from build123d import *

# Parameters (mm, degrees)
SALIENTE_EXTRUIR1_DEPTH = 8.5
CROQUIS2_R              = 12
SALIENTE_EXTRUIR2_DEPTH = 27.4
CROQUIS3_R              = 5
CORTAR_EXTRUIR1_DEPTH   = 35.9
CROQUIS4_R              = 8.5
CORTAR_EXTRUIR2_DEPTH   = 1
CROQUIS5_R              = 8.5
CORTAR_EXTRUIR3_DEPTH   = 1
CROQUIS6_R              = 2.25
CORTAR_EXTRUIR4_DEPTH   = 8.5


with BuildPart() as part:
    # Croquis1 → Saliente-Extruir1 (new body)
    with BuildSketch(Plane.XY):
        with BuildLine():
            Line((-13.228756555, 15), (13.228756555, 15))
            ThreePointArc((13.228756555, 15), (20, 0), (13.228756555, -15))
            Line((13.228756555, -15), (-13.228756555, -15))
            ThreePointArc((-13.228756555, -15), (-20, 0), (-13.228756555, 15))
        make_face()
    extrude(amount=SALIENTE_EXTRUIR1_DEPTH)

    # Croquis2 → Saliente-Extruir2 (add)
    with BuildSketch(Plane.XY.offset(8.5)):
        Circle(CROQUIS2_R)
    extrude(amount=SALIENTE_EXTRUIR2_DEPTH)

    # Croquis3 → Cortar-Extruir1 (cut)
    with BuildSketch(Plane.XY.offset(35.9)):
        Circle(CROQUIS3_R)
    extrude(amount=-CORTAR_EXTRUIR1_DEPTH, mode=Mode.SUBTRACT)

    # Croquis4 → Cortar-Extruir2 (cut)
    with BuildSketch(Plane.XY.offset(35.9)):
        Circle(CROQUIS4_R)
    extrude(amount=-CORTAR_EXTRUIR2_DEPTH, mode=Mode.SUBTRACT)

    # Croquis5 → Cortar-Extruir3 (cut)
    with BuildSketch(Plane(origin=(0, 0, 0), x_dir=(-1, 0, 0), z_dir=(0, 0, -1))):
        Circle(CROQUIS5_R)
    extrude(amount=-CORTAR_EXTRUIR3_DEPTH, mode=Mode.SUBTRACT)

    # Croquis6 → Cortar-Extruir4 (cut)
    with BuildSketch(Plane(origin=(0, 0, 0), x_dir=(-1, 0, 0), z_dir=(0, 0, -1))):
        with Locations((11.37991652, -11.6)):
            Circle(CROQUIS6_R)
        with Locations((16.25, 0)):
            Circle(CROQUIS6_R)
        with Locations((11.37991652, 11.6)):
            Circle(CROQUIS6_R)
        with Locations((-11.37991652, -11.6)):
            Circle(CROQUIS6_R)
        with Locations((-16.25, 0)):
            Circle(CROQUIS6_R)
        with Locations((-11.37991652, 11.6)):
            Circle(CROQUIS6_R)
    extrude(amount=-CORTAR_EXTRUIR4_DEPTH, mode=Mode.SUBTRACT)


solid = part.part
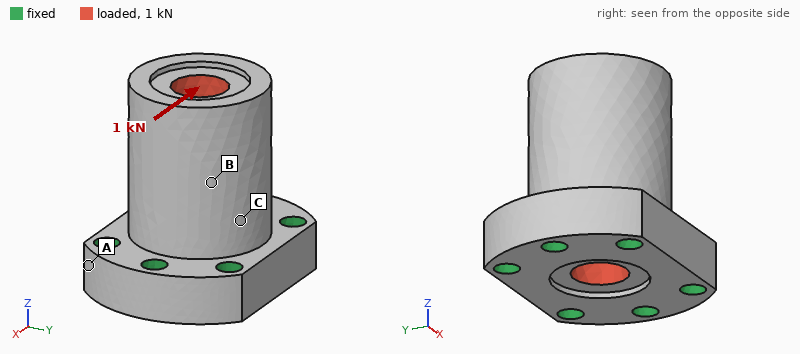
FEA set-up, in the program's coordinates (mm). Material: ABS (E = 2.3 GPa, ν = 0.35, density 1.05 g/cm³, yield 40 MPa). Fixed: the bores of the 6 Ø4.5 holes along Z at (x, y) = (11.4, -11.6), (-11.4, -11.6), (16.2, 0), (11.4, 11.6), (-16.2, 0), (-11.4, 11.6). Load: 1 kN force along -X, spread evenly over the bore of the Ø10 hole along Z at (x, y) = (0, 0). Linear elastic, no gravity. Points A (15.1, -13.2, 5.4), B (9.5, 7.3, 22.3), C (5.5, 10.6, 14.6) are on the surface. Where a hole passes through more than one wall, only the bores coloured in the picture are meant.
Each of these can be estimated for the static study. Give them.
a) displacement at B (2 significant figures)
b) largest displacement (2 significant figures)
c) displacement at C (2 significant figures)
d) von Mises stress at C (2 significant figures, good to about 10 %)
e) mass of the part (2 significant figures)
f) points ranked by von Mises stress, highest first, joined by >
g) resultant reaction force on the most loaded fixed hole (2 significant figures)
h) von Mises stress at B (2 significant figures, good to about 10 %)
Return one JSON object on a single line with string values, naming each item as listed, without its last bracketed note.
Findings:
{"displacement at B": "0.091 mm", "largest displacement": "0.16 mm", "displacement at C": "0.042 mm", "von Mises stress at C": "3.5 MPa", "mass of the part": "18 g", "points ranked by von Mises stress, highest first, joined by >": "C > B > A", "resultant reaction force on the most loaded fixed hole": "330 N", "von Mises stress at B": "2.0 MPa"}
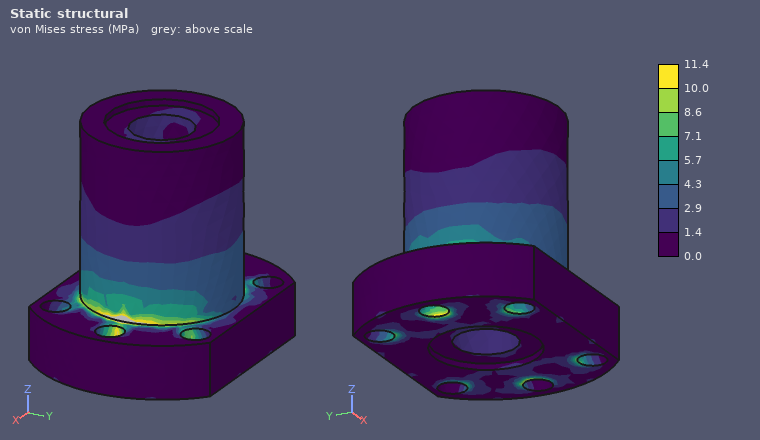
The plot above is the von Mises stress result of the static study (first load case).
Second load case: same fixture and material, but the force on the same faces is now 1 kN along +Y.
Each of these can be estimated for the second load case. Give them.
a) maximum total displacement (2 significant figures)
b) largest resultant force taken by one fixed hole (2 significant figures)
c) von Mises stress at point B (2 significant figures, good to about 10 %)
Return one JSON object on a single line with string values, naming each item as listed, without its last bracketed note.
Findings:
{"maximum total displacement": "0.20 mm", "largest resultant force taken by one fixed hole": "390 N", "von Mises stress at point B": "2.2 MPa"}
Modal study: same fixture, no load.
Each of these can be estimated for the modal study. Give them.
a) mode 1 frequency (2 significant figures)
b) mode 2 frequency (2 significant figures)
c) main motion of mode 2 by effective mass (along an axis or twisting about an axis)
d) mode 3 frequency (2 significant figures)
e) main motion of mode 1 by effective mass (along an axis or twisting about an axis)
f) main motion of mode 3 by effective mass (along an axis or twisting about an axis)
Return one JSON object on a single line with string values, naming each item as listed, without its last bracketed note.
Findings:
{"mode 1 frequency": "3600 Hz", "mode 2 frequency": "4000 Hz", "main motion of mode 2 by effective mass": "along X", "mode 3 frequency": "7400 Hz", "main motion of mode 1 by effective mass": "along Y", "main motion of mode 3 by effective mass": "twisting about Z"}
